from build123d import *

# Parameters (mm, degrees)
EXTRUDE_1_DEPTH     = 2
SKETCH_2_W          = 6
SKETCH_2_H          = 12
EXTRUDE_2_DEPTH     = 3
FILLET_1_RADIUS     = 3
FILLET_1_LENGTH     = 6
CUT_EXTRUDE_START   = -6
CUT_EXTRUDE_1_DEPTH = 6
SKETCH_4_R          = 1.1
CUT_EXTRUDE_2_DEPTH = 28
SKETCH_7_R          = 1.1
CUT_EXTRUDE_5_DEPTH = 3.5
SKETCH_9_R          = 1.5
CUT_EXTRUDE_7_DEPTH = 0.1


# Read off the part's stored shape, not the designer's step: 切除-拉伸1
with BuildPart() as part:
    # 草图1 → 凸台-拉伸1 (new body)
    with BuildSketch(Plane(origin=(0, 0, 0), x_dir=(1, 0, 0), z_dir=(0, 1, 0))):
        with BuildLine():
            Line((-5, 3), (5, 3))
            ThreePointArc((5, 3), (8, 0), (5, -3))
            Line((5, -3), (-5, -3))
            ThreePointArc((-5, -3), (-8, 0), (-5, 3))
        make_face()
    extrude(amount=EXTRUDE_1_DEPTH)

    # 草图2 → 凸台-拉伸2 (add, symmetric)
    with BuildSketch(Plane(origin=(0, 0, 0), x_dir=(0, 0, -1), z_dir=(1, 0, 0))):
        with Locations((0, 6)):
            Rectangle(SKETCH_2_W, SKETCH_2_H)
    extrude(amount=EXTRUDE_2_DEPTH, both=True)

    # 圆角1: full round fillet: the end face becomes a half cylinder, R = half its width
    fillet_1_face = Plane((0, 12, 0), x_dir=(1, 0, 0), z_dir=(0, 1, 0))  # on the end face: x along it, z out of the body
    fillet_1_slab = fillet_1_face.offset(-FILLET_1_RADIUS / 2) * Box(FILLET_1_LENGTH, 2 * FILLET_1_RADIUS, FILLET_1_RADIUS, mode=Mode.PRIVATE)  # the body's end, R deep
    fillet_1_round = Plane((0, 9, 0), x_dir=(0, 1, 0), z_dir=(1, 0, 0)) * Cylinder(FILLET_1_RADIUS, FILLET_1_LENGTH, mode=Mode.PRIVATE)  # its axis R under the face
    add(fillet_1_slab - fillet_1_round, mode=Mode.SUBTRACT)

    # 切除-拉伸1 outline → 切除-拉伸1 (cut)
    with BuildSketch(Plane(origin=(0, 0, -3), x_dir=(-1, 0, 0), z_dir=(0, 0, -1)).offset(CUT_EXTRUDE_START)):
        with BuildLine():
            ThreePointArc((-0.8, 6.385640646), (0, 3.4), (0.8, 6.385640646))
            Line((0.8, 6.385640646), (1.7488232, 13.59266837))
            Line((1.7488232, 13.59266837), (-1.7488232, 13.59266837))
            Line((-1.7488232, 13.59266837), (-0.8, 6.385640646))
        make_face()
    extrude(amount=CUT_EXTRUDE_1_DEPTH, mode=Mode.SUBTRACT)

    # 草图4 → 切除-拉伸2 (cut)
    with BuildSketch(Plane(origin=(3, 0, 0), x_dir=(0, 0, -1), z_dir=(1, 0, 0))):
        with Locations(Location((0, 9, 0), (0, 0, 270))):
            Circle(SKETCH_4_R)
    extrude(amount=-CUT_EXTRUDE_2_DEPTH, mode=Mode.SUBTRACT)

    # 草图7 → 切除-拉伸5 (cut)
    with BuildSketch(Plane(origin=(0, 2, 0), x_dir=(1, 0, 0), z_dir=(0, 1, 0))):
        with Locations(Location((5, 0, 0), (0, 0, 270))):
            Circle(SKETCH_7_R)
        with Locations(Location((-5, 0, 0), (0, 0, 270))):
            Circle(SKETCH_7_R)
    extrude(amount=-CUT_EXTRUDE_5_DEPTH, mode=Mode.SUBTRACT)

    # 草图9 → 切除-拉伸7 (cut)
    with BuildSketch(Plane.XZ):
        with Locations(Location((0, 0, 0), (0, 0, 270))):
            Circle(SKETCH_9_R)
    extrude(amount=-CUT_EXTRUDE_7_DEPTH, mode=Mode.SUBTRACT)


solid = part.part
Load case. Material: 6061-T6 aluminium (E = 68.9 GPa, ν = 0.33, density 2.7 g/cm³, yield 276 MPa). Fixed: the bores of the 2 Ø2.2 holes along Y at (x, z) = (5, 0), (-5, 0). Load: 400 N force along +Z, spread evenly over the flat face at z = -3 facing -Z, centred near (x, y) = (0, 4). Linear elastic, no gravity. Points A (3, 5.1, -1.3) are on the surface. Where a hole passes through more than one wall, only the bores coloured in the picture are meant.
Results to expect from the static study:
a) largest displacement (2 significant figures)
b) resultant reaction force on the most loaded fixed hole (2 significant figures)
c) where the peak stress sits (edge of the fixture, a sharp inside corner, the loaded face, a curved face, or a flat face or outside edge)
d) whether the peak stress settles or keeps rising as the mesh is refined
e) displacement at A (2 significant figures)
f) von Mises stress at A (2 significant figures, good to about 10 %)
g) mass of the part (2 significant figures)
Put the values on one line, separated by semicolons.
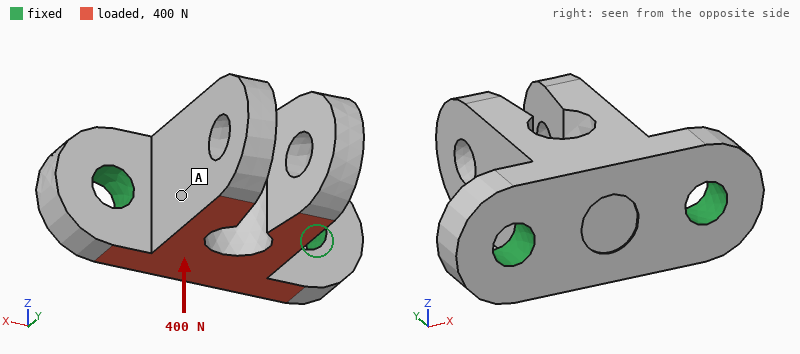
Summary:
31 µm; 200 N; edge of the fixture; keeps rising; 13 µm; 16 MPa; 1.00 g
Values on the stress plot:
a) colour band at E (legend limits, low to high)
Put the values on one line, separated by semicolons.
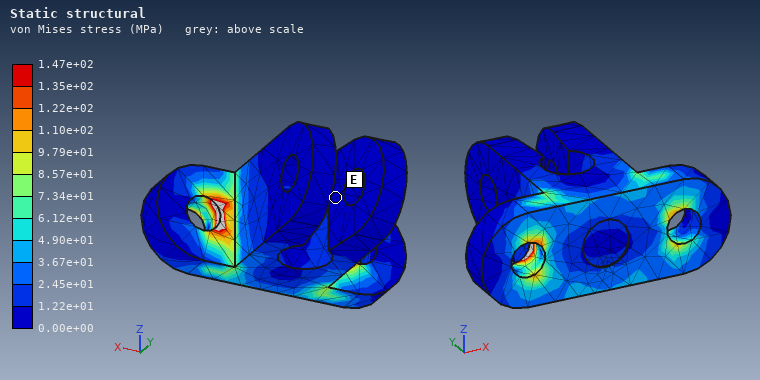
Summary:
0.00e+00 to 1.22e+01 MPa
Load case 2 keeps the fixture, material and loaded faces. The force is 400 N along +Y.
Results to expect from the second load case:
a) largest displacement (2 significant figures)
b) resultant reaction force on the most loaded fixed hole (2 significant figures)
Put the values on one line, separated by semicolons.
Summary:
31 µm; 210 N
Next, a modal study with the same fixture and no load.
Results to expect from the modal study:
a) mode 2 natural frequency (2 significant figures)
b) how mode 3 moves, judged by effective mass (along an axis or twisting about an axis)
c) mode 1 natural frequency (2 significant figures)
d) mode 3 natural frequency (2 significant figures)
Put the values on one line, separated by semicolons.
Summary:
18 kHz; along Z; 18 kHz; 20 kHz
